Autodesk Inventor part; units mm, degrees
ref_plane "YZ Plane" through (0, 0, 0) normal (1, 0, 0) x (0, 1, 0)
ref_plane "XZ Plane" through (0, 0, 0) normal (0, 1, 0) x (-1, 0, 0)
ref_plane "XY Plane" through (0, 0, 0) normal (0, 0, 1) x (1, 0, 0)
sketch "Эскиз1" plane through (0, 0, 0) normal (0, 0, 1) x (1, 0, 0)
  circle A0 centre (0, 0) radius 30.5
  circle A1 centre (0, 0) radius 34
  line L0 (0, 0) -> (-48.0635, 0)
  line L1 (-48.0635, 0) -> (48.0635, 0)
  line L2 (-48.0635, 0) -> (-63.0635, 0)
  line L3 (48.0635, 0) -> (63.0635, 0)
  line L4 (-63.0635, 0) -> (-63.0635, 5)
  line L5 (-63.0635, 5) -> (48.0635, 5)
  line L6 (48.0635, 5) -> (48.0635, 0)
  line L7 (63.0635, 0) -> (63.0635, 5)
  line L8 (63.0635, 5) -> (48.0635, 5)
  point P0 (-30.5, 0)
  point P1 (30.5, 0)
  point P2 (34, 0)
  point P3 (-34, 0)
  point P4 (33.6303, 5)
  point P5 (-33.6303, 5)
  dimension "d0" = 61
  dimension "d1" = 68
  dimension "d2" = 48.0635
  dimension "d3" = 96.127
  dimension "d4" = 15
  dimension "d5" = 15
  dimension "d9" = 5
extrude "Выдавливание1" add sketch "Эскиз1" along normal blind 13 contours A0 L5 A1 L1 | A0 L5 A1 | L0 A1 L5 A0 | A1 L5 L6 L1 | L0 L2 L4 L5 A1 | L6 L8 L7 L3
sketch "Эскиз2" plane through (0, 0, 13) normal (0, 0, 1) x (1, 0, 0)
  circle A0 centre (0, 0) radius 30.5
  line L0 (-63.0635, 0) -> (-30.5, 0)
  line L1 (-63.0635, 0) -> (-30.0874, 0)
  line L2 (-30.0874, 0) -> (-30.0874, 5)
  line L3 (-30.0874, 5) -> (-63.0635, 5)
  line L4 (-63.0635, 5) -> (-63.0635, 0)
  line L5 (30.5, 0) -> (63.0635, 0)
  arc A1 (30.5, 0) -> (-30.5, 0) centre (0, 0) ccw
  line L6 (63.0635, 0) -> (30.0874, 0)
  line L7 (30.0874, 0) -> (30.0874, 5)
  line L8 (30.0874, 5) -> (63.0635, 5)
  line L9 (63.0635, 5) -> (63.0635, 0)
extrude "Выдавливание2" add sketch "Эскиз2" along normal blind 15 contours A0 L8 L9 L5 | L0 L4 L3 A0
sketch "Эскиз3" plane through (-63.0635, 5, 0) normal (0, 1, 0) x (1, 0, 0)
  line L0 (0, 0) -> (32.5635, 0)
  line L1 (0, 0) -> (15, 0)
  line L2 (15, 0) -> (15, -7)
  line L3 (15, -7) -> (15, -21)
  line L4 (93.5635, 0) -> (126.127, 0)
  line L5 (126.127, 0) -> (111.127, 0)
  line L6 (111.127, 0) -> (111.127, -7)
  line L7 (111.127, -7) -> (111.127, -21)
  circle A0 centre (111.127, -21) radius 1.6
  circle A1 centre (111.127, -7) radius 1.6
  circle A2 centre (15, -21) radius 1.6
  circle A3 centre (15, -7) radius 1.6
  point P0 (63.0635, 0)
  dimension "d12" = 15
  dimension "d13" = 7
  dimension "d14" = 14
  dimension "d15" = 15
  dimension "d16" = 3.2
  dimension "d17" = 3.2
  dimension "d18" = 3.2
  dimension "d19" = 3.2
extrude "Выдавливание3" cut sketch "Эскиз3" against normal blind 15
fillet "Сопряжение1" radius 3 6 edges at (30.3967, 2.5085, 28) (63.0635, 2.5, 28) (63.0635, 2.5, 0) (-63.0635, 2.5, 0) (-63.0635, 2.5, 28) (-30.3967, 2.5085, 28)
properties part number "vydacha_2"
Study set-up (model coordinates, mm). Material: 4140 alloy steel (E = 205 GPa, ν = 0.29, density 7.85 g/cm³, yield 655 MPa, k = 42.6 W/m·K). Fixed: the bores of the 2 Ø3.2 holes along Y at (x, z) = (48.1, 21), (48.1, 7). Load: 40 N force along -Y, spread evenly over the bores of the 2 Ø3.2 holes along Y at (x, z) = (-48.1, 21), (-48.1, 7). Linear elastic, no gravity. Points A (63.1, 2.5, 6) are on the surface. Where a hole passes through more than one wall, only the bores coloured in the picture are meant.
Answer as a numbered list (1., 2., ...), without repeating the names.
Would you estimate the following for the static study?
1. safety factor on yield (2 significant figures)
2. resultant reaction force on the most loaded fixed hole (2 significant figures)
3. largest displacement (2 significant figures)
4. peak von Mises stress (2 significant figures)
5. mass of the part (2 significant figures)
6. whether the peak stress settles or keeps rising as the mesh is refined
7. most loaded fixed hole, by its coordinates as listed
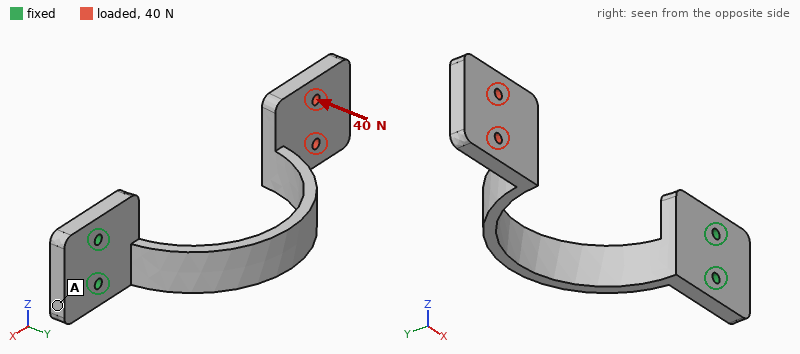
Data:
1. 4.6
2. 27 N
3. 1.6 mm
4. 140 MPa
5. 100 g
6. settles
7. (48.1, 21)
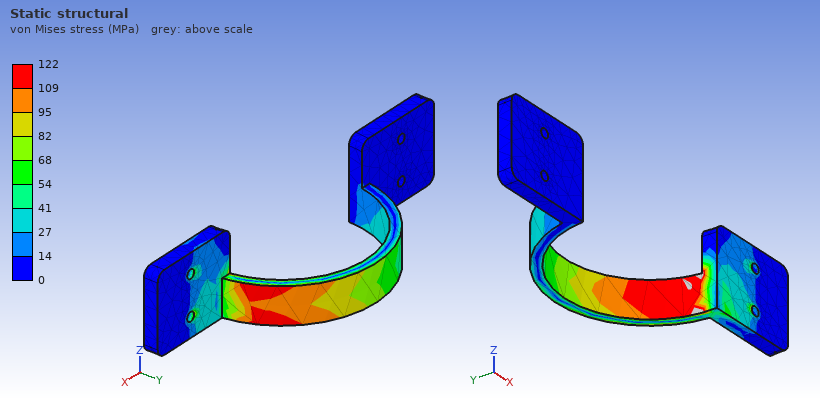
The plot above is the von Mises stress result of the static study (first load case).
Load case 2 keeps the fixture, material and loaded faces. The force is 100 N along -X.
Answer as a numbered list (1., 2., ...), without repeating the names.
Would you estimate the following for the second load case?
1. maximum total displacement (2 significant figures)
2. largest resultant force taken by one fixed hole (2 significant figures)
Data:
1. 1.3 mm
2. 53 N
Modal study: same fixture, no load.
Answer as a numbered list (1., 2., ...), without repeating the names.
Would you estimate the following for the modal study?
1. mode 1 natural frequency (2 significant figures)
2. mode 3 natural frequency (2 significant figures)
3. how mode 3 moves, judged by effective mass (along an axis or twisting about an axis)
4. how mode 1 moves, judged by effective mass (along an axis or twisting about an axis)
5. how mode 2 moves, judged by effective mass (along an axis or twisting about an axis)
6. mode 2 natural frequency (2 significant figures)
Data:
1. 140 Hz
2. 540 Hz
3. along X
4. along Y
5. along Z
6. 210 Hz
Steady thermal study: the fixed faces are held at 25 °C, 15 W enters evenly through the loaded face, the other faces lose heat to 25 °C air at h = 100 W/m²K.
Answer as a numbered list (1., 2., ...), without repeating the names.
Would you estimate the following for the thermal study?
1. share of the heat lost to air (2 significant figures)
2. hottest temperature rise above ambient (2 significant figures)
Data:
1. 99 %
2. 63 K
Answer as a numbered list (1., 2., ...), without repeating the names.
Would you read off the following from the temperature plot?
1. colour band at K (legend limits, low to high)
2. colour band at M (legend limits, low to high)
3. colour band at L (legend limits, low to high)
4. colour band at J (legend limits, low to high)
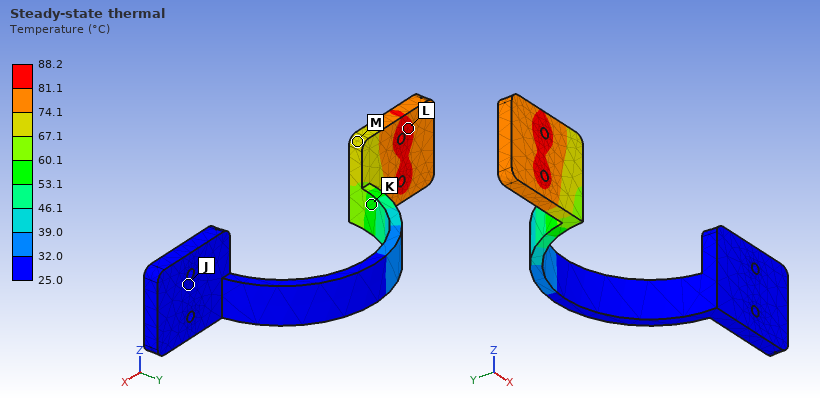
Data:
1. 53.1 to 60.1 °C
2. 67.1 to 74.1 °C
3. 81.1 to 88.2 °C
4. 25.0 to 32.0 °C
